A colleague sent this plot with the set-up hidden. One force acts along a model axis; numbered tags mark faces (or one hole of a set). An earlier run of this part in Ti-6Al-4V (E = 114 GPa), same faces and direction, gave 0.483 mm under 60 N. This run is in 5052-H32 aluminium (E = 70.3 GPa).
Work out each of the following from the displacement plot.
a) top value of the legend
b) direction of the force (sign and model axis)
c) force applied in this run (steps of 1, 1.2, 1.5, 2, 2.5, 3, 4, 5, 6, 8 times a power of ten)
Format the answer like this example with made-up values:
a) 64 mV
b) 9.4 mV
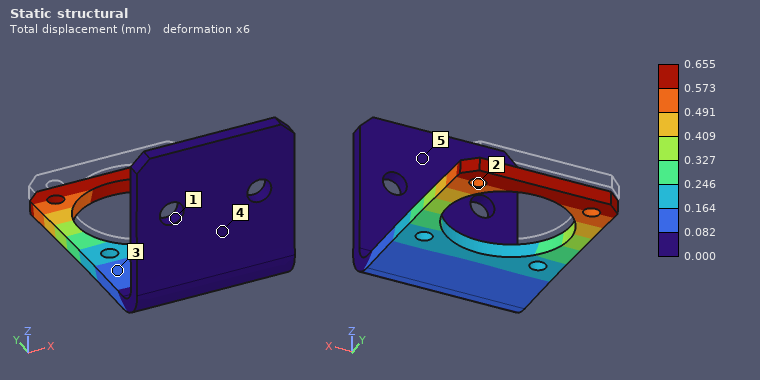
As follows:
a) 0.655 mm
b) -Z
c) 50 N
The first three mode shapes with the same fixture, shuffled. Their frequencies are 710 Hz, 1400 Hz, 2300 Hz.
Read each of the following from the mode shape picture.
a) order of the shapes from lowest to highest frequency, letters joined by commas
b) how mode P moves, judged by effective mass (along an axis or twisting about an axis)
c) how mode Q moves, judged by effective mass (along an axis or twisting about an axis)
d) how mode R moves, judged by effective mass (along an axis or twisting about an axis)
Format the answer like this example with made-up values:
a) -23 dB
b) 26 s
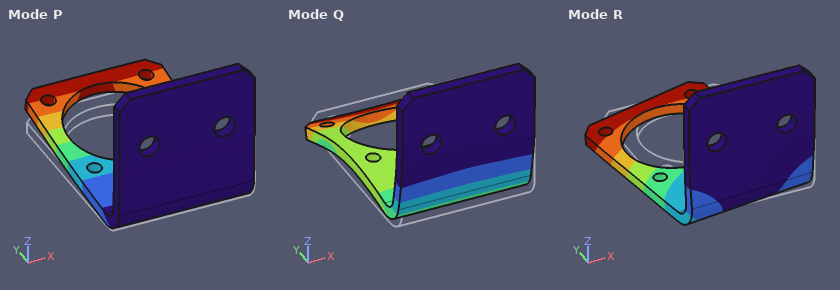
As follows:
a) P, R, Q
b) along Z
c) along Y
d) along X
